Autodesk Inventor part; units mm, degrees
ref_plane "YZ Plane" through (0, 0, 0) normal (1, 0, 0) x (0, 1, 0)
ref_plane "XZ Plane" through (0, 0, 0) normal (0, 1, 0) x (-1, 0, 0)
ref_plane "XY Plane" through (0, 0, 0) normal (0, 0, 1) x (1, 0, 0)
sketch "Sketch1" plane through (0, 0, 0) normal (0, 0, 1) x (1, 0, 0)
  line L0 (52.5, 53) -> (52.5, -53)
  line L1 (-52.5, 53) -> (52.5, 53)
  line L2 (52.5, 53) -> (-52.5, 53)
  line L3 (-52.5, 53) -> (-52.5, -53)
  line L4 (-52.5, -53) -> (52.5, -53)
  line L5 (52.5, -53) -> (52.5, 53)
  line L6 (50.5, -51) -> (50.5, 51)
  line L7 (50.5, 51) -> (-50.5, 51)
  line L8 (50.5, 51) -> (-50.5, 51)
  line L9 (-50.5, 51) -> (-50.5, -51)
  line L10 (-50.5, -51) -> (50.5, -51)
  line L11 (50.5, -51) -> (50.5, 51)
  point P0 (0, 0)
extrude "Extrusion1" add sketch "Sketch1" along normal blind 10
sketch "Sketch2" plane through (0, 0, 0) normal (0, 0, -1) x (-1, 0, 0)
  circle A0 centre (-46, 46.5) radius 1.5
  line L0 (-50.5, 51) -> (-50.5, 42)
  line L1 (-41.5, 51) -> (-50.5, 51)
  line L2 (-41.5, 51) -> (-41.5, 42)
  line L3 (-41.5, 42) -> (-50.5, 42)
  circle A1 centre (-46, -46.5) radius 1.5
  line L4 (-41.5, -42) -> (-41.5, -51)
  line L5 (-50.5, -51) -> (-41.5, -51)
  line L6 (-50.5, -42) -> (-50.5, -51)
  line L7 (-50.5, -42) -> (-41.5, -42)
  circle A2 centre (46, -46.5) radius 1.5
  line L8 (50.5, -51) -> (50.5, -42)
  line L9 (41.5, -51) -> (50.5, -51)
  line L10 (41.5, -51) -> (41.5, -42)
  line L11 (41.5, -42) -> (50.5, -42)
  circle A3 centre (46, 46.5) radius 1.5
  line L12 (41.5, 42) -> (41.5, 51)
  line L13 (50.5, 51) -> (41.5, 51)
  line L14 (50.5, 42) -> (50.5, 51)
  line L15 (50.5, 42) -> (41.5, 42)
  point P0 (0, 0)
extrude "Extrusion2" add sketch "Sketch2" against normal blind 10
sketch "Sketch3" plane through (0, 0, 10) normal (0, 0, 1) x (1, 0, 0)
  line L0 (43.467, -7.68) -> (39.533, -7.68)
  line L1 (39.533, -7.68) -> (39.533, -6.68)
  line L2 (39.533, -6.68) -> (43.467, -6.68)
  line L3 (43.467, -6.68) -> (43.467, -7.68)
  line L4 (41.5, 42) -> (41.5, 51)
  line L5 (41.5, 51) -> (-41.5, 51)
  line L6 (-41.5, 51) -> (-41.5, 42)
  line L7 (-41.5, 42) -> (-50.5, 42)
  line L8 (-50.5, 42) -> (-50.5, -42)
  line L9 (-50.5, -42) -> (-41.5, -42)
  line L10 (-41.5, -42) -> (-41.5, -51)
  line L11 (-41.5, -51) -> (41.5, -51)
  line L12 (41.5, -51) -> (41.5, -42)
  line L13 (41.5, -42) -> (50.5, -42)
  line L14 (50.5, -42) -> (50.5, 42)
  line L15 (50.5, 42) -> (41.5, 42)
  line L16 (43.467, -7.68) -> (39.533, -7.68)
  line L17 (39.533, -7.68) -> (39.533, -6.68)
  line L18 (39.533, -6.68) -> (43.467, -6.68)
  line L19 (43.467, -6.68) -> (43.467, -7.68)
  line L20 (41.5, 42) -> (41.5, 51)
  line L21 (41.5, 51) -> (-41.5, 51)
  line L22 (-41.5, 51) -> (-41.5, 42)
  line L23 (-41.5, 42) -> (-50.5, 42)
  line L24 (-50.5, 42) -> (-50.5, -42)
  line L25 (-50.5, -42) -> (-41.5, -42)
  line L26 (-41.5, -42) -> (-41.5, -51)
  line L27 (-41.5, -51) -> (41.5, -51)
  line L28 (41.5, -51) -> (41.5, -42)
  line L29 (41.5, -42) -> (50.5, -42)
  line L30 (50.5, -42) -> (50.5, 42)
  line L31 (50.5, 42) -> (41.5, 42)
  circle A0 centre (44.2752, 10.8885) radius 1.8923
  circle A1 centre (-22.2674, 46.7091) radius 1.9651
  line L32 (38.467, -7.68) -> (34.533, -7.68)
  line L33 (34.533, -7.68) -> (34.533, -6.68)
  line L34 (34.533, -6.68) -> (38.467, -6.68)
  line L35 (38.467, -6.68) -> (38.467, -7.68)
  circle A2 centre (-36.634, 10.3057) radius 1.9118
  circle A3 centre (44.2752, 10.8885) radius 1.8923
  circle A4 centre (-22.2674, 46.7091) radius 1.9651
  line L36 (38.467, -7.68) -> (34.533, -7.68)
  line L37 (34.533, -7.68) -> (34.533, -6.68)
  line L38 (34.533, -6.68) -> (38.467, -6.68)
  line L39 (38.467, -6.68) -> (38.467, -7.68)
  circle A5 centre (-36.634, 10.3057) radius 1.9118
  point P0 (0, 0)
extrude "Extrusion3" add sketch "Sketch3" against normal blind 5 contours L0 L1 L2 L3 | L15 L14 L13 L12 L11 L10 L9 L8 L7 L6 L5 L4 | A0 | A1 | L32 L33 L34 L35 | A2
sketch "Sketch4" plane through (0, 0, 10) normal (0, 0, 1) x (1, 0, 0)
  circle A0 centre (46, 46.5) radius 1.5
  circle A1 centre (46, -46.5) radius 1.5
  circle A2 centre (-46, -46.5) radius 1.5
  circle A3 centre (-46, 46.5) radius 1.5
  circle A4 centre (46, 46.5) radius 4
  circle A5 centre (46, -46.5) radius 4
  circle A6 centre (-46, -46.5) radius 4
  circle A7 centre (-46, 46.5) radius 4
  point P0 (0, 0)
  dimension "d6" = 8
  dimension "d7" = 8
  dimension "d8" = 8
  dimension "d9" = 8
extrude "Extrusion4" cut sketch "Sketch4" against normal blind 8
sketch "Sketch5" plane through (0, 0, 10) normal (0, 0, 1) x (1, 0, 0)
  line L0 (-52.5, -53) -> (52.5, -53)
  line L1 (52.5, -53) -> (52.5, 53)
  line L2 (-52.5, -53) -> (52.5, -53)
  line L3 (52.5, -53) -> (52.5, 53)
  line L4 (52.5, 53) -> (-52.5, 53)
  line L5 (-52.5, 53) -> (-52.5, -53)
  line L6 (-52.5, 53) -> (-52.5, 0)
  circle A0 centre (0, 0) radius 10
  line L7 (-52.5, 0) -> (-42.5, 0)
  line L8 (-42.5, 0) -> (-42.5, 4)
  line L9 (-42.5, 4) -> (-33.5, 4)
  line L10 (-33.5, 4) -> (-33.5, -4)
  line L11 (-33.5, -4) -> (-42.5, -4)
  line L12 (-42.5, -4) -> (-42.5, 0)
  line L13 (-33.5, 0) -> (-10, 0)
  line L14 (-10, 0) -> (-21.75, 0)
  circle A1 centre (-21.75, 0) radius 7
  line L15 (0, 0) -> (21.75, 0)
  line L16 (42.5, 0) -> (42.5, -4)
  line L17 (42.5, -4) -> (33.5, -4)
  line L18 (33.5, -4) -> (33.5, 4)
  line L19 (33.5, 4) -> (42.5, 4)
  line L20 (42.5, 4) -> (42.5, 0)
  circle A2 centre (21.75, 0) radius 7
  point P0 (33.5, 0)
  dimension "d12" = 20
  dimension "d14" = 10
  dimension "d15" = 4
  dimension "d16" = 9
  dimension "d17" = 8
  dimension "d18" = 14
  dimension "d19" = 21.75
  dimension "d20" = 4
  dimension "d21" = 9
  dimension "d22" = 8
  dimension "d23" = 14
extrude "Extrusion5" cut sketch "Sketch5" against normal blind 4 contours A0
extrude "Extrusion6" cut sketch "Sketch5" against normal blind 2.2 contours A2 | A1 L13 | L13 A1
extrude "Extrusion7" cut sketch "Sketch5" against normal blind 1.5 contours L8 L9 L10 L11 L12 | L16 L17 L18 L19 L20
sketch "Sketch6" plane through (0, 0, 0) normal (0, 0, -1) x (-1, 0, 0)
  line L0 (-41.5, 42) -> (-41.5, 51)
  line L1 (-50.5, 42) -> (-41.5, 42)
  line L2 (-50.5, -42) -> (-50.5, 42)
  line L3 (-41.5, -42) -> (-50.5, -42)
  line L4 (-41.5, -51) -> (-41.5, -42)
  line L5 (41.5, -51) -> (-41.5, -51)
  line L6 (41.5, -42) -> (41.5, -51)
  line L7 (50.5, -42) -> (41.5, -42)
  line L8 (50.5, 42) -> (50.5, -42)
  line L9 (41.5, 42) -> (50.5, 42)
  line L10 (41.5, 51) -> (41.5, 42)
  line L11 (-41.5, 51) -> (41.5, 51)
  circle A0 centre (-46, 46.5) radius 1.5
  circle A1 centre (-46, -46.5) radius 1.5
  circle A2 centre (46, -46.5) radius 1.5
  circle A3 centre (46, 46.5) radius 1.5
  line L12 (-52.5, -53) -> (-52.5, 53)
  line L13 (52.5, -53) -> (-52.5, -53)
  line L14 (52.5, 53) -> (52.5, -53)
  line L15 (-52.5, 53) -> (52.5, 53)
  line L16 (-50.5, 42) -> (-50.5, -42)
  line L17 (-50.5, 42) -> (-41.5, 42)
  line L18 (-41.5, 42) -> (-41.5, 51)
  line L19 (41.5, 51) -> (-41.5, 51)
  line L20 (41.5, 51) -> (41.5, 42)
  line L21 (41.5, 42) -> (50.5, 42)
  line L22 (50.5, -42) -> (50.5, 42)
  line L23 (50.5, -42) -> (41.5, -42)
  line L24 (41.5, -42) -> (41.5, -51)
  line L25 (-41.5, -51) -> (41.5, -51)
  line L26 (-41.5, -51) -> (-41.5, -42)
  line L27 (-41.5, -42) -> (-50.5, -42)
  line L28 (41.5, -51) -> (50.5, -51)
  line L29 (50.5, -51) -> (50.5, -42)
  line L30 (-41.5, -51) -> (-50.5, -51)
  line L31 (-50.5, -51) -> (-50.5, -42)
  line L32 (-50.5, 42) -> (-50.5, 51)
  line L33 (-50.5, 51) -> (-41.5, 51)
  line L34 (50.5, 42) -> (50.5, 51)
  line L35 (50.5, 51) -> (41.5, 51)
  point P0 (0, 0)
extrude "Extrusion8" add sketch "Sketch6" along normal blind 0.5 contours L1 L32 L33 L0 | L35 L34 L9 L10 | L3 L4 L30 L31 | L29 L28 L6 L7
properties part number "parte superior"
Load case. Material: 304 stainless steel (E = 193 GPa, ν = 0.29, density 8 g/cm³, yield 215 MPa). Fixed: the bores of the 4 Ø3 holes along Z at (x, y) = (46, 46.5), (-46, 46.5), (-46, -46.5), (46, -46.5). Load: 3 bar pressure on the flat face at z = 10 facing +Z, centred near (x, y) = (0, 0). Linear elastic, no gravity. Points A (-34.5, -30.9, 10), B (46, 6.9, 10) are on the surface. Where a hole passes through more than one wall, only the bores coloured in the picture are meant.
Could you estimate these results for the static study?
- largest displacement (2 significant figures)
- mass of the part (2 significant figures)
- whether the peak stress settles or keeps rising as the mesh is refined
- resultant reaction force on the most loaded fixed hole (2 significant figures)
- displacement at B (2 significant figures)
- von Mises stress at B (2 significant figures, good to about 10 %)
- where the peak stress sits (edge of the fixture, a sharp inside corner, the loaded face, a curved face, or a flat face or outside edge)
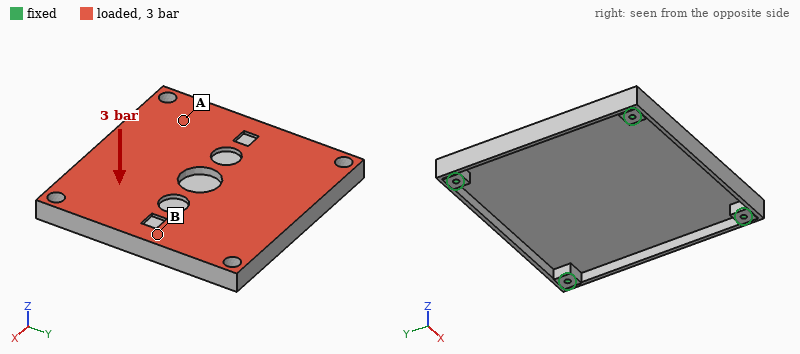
88 µm
460 g
keeps rising
1.4 kN
38 µm
34 MPa
edge of the fixture
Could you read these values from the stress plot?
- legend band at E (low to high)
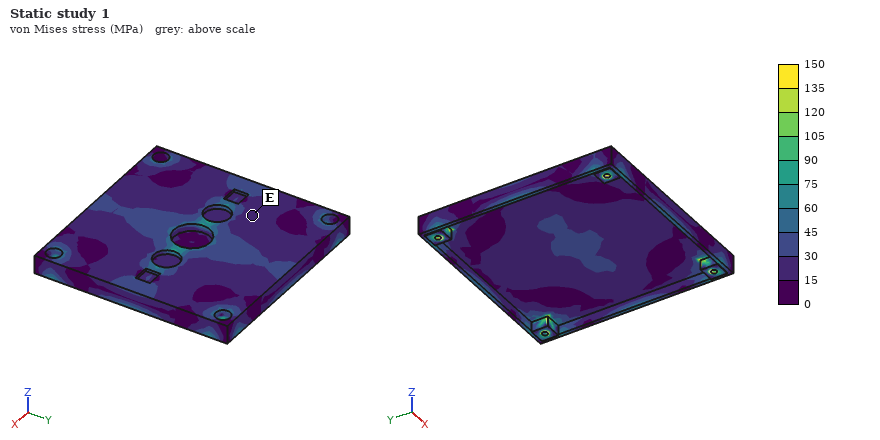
15 to 30 MPa
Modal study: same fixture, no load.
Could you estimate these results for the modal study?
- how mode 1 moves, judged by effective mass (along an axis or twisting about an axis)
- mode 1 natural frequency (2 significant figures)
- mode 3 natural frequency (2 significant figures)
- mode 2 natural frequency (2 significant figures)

along Z
1800 Hz
3300 Hz
3200 Hz
